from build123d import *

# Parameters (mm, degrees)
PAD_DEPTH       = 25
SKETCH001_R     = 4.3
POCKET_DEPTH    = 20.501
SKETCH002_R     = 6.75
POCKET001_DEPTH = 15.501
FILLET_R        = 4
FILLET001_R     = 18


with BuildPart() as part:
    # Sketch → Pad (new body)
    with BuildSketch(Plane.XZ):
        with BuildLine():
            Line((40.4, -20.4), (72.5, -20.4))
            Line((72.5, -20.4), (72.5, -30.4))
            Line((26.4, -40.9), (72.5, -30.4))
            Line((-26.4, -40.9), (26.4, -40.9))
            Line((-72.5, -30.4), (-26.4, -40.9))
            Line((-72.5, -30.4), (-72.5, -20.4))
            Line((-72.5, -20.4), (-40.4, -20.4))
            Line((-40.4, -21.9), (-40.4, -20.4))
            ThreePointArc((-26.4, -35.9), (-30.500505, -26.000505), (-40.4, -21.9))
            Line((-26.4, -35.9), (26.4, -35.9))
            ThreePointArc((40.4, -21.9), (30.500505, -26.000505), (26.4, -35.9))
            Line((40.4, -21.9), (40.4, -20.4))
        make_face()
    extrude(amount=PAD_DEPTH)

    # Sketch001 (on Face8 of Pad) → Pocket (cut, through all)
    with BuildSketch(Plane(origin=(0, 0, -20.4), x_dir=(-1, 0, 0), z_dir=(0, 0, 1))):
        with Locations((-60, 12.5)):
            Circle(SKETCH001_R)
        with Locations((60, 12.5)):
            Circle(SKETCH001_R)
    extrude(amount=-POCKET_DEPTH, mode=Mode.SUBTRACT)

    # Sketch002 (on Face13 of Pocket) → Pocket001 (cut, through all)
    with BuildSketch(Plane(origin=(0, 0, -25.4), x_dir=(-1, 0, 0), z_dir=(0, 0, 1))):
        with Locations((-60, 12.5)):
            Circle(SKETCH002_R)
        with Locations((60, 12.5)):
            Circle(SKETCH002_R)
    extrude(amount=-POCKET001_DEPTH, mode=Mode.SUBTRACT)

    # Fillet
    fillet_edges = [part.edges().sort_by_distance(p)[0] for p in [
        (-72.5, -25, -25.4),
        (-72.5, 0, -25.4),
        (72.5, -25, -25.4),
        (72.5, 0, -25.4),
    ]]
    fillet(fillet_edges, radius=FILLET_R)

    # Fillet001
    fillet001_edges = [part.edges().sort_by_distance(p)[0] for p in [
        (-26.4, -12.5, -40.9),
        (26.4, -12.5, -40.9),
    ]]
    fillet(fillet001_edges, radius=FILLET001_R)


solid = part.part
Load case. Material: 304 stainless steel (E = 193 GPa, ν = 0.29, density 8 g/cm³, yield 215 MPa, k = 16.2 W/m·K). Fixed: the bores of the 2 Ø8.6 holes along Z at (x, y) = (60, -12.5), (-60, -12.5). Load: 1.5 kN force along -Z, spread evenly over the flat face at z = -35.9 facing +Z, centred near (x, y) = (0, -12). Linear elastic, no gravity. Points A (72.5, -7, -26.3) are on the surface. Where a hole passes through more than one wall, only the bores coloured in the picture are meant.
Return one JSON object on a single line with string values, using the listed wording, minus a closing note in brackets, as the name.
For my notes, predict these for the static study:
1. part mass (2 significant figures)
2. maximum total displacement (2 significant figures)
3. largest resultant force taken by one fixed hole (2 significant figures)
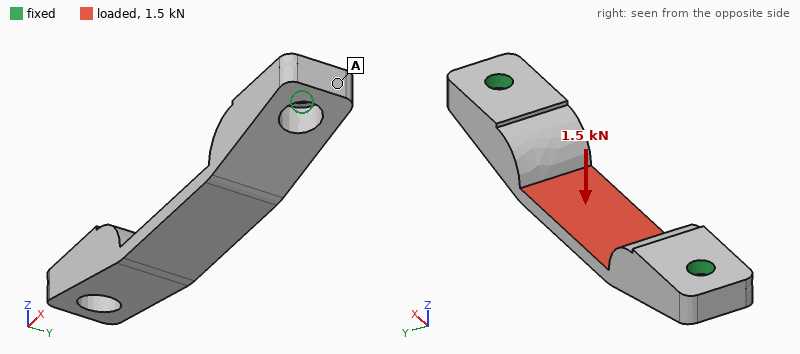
{"part mass": "280 g", "maximum total displacement": "26 µm", "largest resultant force taken by one fixed hole": "1.8 kN"}
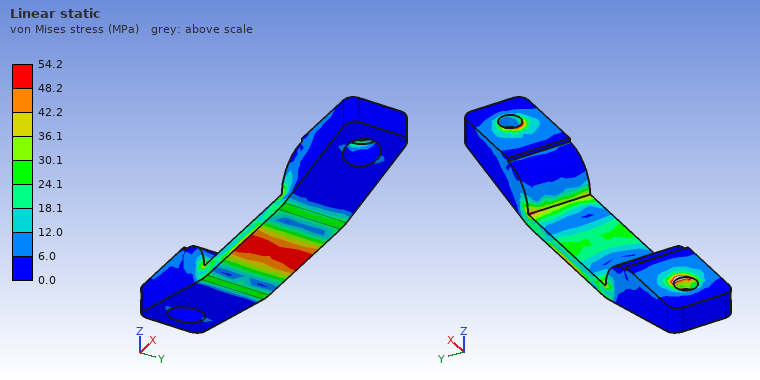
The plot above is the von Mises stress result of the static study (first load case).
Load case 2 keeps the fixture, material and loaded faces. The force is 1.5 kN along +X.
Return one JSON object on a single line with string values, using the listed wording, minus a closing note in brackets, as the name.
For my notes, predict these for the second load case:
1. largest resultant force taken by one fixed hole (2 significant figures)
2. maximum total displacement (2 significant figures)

{"largest resultant force taken by one fixed hole": "750 N", "maximum total displacement": "9.9 µm"}
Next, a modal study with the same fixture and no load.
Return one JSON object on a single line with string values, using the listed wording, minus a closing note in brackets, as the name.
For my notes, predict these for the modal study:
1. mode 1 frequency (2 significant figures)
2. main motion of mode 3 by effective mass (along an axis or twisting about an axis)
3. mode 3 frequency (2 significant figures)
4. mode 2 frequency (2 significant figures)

{"mode 1 frequency": "4700 Hz", "main motion of mode 3 by effective mass": "along Z", "mode 3 frequency": "5600 Hz", "mode 2 frequency": "4700 Hz"}
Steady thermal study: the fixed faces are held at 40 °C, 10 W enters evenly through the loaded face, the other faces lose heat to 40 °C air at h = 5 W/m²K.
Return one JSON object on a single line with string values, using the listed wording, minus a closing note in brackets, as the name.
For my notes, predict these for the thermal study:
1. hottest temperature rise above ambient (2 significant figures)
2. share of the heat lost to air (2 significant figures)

{"hottest temperature rise above ambient": "70 K", "share of the heat lost to air": "12 %"}
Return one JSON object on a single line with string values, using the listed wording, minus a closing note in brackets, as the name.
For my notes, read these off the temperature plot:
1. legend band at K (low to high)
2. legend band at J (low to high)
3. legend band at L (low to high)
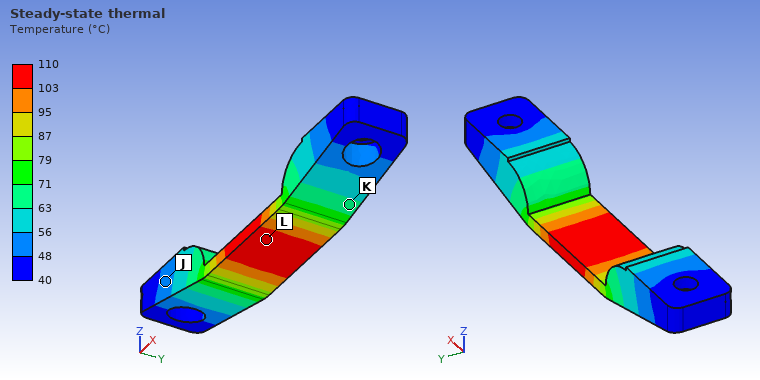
{"legend band at K": "63 to 71 °C", "legend band at J": "48 to 56 °C", "legend band at L": "103 to 110 °C"}
